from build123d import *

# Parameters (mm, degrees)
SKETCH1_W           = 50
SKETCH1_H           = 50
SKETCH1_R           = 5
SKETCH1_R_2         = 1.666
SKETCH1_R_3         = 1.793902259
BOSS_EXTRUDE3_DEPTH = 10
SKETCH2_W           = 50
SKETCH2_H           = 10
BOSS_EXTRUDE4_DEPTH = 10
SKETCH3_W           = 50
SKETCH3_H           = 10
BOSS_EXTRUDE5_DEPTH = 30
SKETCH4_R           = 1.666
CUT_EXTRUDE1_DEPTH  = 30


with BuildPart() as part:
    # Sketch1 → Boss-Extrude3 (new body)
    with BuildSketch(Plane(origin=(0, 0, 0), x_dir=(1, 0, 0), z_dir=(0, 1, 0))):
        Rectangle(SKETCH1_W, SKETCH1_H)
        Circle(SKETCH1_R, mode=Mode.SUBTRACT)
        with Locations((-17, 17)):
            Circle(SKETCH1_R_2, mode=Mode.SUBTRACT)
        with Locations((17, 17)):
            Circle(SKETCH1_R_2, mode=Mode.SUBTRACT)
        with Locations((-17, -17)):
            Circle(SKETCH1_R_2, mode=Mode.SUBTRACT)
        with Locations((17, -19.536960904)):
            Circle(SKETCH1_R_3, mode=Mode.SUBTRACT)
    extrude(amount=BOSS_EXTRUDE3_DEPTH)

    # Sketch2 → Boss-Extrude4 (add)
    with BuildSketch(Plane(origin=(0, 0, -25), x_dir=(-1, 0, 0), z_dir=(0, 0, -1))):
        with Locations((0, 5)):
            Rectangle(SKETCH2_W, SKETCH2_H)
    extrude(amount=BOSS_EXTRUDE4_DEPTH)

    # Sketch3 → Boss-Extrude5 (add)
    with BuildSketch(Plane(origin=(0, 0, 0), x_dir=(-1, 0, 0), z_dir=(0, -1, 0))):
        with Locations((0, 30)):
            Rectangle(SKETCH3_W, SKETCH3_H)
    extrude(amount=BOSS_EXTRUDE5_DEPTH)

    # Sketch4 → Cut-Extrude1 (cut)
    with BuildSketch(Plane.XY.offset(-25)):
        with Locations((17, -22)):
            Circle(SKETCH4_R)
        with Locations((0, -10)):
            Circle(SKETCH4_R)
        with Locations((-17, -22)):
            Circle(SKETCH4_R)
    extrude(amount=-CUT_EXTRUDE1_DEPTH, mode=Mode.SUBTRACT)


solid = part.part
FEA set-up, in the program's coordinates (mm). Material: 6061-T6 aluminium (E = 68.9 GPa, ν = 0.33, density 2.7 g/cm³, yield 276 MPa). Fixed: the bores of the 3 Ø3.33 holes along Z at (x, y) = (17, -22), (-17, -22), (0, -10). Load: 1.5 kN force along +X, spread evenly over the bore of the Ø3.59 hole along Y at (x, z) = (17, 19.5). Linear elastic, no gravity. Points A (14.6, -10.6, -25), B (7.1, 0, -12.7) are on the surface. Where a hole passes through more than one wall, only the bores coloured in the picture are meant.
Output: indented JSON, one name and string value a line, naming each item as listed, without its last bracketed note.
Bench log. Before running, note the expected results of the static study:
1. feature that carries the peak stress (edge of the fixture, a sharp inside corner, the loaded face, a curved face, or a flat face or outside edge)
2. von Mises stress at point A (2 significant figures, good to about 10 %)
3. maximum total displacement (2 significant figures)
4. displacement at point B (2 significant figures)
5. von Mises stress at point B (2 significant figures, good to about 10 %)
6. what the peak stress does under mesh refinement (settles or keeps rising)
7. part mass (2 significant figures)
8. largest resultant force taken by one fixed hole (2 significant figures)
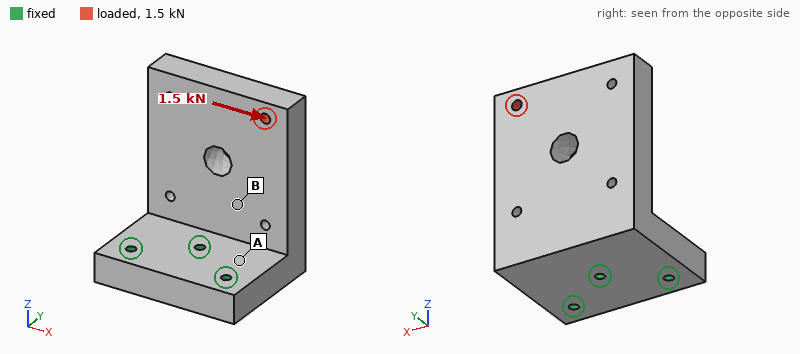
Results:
{
  "feature that carries the peak stress": "edge of the fixture",
  "von Mises stress at point A": "42 MPa",
  "maximum total displacement": "0.16 mm",
  "displacement at point B": "0.049 mm",
  "von Mises stress at point B": "17 MPa",
  "what the peak stress does under mesh refinement": "keeps rising",
  "part mass": "120 g",
  "largest resultant force taken by one fixed hole": "1.6 kN"
}
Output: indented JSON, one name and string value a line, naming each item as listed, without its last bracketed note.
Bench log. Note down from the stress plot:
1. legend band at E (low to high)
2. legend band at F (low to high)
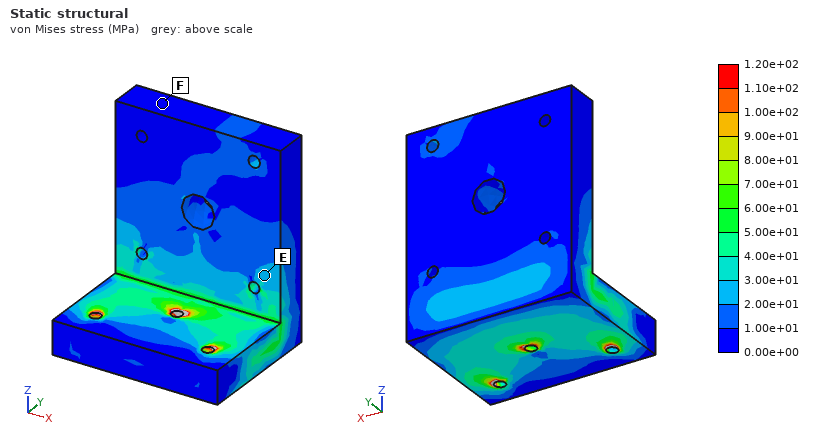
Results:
{
  "legend band at E": "2.00e+01 to 3.00e+01 MPa",
  "legend band at F": "0.00e+00 to 1.00e+01 MPa"
}
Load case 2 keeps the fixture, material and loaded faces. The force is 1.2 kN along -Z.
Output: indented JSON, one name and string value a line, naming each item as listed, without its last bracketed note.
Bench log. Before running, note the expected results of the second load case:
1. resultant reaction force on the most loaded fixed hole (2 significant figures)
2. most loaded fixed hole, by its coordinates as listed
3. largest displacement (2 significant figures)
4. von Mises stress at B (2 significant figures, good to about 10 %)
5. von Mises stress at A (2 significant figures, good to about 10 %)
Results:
{
  "resultant reaction force on the most loaded fixed hole": "1.4 kN",
  "most loaded fixed hole, by its coordinates as listed": "(0, -10)",
  "largest displacement": "73 µm",
  "von Mises stress at B": "5.7 MPa",
  "von Mises stress at A": "19 MPa"
}
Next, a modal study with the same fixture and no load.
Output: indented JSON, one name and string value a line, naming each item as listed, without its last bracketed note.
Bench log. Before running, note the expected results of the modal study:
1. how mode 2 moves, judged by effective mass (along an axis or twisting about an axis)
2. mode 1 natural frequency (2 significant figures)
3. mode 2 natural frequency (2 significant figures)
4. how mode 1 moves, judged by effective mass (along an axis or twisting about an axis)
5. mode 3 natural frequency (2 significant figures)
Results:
{
  "how mode 2 moves, judged by effective mass": "along X",
  "mode 1 natural frequency": "1800 Hz",
  "mode 2 natural frequency": "2900 Hz",
  "how mode 1 moves, judged by effective mass": "along Y",
  "mode 3 natural frequency": "5800 Hz"
}
